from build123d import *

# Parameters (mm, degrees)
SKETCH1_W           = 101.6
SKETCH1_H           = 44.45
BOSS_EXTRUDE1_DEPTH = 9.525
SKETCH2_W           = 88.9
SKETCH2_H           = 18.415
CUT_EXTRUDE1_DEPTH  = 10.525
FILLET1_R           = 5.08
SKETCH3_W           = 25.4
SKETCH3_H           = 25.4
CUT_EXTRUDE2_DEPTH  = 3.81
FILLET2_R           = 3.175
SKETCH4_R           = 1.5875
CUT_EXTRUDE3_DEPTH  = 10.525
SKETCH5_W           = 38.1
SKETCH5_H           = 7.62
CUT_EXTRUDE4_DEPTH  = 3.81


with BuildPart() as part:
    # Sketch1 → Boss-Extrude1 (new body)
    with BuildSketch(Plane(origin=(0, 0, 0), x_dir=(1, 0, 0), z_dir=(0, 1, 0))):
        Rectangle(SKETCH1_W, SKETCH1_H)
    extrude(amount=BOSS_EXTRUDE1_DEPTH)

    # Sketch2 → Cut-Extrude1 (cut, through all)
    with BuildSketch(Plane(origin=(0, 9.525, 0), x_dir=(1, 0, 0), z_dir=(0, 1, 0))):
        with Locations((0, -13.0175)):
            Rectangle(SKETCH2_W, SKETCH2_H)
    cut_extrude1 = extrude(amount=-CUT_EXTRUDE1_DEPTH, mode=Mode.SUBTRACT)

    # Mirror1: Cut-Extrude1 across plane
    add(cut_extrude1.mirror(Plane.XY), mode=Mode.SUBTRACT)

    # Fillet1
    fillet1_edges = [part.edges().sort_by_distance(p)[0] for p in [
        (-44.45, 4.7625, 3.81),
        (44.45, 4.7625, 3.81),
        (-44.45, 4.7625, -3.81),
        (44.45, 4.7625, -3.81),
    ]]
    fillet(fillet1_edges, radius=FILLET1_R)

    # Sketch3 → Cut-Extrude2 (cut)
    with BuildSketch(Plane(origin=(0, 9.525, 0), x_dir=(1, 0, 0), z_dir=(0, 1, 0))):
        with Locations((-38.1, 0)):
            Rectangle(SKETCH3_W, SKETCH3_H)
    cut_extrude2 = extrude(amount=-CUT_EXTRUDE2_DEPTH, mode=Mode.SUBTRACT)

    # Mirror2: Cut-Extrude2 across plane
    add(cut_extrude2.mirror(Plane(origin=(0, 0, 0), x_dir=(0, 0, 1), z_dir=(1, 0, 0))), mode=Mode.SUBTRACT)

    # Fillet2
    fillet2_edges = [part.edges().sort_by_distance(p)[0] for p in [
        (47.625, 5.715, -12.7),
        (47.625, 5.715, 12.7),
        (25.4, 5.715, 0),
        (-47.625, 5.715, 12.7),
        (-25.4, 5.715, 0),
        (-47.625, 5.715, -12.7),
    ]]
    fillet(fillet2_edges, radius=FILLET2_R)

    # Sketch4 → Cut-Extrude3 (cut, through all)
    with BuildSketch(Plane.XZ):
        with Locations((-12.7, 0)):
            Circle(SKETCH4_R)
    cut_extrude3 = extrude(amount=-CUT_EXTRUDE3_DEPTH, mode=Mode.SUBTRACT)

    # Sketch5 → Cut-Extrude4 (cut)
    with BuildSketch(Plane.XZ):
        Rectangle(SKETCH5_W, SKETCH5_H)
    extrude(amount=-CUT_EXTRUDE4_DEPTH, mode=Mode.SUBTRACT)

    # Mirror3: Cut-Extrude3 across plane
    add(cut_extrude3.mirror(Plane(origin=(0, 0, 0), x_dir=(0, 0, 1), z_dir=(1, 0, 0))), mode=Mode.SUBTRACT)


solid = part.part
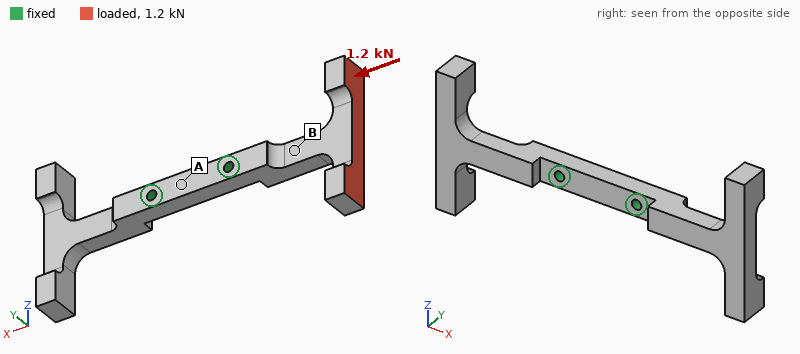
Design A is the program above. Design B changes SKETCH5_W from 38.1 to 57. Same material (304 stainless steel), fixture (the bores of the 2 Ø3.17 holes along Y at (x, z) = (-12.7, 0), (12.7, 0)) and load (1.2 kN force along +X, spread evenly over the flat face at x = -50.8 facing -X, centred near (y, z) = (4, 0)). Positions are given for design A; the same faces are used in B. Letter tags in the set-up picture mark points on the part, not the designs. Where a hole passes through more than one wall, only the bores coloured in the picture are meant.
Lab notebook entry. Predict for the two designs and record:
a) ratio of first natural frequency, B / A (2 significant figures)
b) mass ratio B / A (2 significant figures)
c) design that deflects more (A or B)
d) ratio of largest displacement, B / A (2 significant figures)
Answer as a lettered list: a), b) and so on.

a) 0.53
b) 0.94
c) B
d) 3.4
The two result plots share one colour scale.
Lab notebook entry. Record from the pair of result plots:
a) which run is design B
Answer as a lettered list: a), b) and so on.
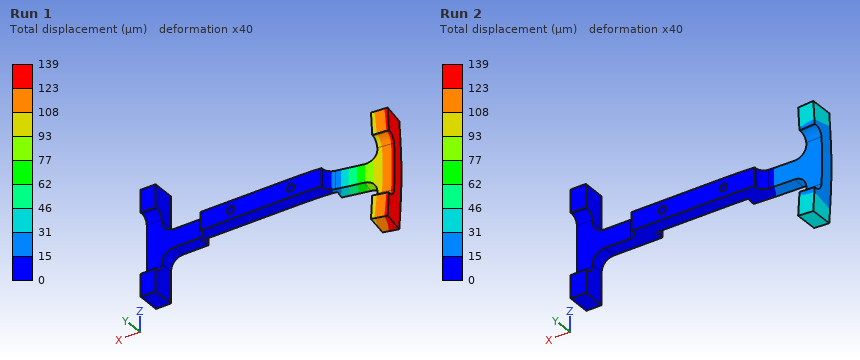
a) Run 1
